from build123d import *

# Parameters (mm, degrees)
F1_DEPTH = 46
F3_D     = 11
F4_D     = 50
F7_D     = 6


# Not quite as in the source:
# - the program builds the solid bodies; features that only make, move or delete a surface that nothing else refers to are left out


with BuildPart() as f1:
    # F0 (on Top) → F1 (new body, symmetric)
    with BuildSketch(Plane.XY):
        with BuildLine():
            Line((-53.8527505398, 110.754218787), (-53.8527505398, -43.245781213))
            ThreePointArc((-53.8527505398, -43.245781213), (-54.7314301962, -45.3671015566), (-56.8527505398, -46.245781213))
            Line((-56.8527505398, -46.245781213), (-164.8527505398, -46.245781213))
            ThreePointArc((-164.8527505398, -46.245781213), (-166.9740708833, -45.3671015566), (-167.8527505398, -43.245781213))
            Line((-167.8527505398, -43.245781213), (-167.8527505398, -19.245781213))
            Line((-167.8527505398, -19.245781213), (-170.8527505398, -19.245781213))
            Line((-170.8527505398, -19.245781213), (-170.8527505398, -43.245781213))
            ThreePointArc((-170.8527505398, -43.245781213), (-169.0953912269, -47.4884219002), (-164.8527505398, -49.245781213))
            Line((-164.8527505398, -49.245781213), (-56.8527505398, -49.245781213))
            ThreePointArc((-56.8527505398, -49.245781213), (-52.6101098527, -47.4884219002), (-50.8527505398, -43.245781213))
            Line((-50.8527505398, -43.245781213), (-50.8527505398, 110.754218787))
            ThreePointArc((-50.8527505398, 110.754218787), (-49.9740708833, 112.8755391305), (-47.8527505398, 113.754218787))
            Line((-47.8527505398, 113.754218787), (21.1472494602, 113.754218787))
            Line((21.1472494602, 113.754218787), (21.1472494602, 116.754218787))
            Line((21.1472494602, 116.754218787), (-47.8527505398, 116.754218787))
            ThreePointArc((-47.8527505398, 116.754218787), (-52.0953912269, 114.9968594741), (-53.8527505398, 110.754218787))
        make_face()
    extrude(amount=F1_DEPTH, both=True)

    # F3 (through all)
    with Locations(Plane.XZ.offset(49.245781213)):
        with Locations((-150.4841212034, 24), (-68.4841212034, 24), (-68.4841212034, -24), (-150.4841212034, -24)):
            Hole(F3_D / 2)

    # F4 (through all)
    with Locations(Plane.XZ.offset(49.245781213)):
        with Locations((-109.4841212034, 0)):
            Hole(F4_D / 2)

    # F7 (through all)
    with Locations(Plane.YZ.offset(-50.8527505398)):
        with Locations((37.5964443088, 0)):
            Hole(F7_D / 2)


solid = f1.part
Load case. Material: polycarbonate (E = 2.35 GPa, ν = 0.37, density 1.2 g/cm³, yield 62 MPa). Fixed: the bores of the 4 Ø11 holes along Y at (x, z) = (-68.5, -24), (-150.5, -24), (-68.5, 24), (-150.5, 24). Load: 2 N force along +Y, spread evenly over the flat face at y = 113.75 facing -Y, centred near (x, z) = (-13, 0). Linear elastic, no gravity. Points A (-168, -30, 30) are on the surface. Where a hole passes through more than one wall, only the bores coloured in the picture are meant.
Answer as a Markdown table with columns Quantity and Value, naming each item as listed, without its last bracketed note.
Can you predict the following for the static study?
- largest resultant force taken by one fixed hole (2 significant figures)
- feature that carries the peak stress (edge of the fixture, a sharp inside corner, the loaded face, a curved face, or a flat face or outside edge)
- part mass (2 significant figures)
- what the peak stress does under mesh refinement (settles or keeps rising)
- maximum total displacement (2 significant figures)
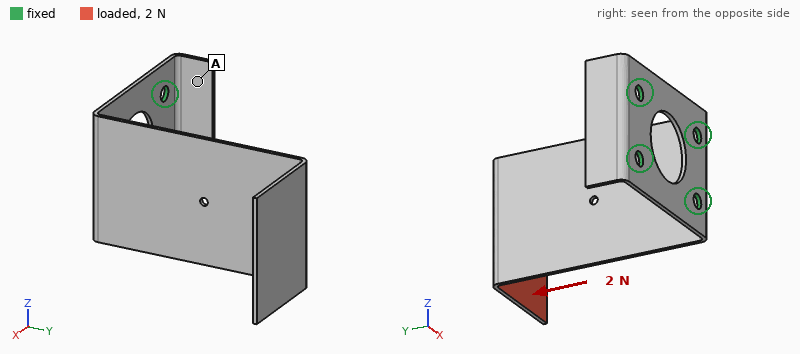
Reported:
| Quantity | Value |
|---|---|
| largest resultant force taken by one fixed hole | 1.1 N |
| feature that carries the peak stress | edge of the fixture |
| part mass | 120 g |
| what the peak stress does under mesh refinement | keeps rising |
| maximum total displacement | 3.2 mm |
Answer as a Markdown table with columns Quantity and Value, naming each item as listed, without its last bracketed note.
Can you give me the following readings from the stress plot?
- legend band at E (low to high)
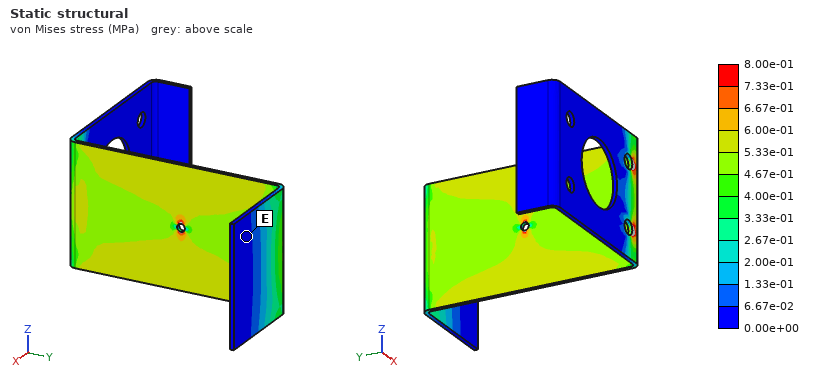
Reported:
| Quantity | Value |
|---|---|
| legend band at E | 0.00e+00 to 6.67e-02 MPa |
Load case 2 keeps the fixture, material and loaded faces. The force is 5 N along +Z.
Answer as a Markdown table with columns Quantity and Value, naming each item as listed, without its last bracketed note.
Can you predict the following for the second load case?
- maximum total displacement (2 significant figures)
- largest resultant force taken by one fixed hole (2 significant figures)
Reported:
| Quantity | Value |
|---|---|
| maximum total displacement | 3.2 mm |
| largest resultant force taken by one fixed hole | 16 N |
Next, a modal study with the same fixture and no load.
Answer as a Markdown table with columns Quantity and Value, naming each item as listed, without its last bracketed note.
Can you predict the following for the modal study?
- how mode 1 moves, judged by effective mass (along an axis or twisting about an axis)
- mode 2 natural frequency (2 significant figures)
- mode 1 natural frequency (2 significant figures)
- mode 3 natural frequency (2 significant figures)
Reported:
| Quantity | Value |
|---|---|
| how mode 1 moves, judged by effective mass | along X |
| mode 2 natural frequency | 43 Hz |
| mode 1 natural frequency | 14 Hz |
| mode 3 natural frequency | 65 Hz |
